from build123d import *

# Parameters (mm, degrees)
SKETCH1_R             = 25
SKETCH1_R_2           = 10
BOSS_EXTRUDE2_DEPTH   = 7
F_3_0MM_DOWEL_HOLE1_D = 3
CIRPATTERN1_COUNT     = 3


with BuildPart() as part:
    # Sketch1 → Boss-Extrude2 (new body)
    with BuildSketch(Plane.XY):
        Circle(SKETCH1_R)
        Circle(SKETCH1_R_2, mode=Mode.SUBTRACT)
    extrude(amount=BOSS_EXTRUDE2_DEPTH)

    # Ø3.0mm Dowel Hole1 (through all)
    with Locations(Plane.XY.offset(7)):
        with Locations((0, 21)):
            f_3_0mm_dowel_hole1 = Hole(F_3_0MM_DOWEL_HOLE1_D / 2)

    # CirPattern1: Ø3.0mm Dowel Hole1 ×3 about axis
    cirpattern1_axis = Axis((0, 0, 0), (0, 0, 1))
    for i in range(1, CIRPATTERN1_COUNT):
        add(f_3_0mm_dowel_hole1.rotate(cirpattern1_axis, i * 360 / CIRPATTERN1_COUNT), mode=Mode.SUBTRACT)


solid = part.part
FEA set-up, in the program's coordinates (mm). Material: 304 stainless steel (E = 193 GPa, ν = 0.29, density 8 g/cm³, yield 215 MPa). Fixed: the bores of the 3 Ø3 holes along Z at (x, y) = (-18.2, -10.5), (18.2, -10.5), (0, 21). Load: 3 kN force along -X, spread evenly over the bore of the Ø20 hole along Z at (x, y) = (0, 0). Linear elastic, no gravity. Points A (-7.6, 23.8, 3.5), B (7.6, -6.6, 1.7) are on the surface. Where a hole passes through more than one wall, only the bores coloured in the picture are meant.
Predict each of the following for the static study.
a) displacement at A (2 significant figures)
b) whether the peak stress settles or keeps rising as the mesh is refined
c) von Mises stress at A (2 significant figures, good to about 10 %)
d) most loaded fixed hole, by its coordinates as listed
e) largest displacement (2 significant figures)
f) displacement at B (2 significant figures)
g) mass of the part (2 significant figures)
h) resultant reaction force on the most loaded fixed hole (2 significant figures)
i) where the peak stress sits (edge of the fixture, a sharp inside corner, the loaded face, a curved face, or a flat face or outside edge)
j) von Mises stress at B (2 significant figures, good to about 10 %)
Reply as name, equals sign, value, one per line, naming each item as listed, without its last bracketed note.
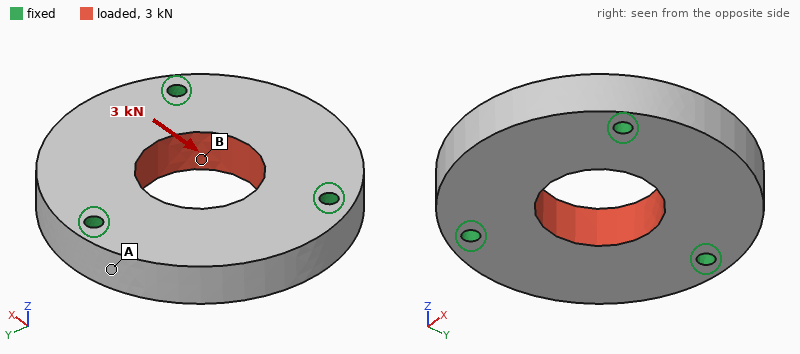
displacement at A = 0.33 µm
whether the peak stress settles or keeps rising as the mesh is refined = keeps rising
von Mises stress at A = 5.9 MPa
most loaded fixed hole, by its coordinates as listed = (0, 21)
largest displacement = 1.5 µm
displacement at B = 0.78 µm
mass of the part = 91 g
resultant reaction force on the most loaded fixed hole = 1.1 kN
where the peak stress sits = edge of the fixture
von Mises stress at B = 14 MPa
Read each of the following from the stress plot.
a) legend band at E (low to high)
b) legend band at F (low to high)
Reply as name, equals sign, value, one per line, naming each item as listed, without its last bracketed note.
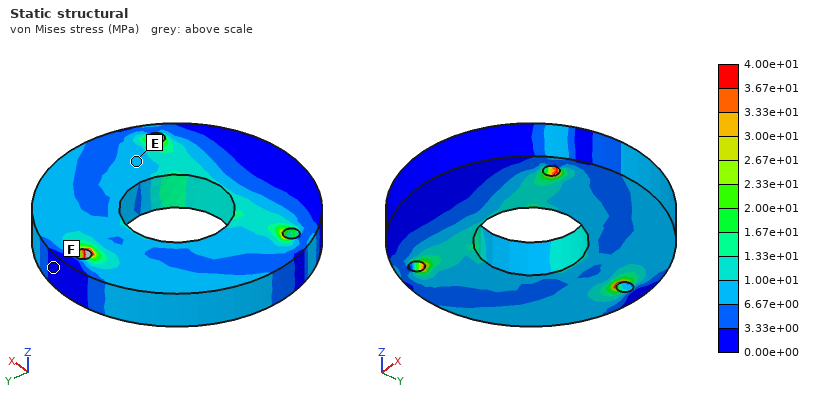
legend band at E = 6.67e+00 to 1.00e+01 MPa
legend band at F = 0.00e+00 to 3.33e+00 MPa
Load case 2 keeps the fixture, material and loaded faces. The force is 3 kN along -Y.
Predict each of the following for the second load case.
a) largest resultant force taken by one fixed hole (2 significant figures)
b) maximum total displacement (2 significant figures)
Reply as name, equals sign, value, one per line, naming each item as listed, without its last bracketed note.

largest resultant force taken by one fixed hole = 1.1 kN
maximum total displacement = 1.7 µm
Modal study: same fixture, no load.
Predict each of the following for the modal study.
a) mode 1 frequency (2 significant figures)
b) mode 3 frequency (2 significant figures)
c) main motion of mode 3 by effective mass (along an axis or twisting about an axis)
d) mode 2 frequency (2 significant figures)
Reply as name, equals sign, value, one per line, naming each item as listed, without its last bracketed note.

mode 1 frequency = 15 kHz
mode 3 frequency = 17 kHz
main motion of mode 3 by effective mass = along Z
mode 2 frequency = 15 kHz
